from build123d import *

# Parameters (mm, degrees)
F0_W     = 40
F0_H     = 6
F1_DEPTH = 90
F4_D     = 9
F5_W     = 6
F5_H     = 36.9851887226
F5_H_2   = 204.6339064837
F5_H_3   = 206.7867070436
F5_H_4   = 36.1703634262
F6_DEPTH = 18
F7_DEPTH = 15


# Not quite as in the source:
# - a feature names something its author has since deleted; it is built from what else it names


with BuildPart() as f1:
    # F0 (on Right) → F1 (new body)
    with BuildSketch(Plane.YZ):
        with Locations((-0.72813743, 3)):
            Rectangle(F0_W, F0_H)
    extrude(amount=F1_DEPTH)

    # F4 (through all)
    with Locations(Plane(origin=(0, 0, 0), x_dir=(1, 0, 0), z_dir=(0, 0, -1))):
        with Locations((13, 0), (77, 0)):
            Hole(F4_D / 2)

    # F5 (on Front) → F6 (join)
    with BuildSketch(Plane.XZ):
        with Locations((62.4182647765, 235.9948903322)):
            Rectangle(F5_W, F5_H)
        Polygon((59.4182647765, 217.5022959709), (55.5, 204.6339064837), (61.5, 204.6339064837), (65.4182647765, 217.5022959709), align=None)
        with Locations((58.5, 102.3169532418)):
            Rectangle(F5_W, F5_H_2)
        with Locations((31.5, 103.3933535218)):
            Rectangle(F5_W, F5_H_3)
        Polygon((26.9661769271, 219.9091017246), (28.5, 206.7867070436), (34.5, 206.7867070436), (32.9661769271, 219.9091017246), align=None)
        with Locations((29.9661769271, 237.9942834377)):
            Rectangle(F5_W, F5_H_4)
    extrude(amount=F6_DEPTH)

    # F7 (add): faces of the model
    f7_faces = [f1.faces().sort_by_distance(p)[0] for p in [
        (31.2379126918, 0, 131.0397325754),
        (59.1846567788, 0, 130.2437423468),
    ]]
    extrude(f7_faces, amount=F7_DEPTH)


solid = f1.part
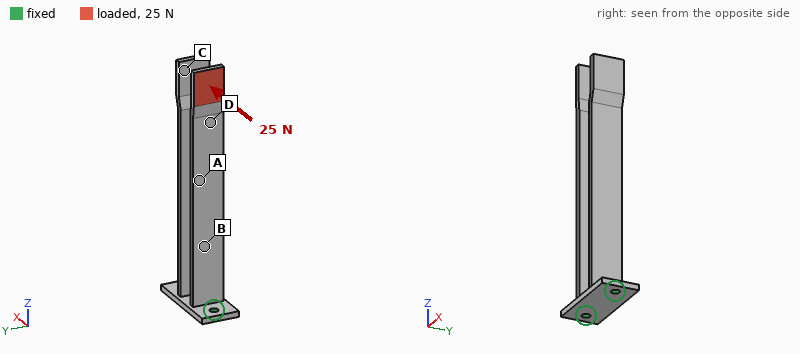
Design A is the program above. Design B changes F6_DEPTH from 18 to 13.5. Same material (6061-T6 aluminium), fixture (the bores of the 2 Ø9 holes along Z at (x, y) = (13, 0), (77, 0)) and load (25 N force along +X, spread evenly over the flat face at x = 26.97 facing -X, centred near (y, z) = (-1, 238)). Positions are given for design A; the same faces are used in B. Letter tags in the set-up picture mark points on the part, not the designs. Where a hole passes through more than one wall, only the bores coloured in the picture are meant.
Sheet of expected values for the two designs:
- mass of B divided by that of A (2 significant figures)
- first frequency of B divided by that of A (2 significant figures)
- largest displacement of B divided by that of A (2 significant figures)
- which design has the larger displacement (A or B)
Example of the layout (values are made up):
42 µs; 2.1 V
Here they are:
0.89; 1.0; 1.2; B
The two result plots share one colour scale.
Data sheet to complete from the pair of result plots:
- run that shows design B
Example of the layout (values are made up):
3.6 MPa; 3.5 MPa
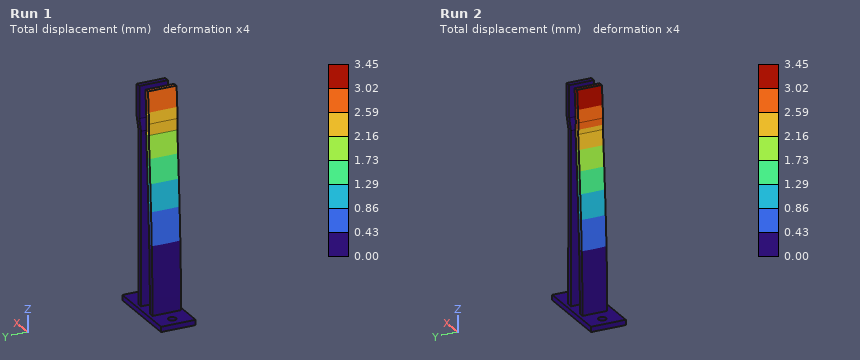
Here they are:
Run 2
